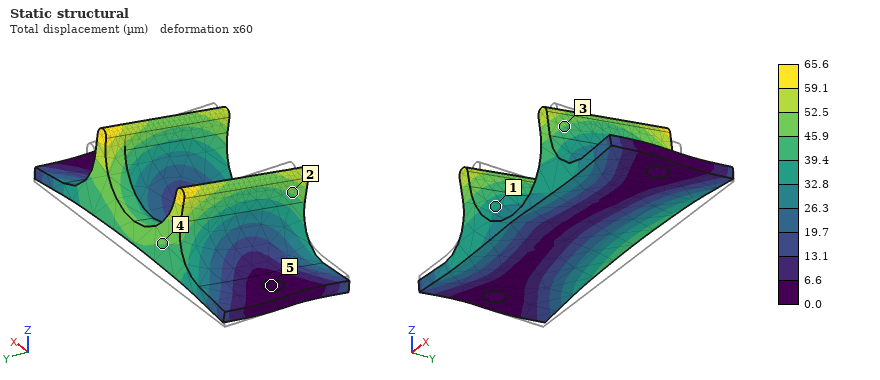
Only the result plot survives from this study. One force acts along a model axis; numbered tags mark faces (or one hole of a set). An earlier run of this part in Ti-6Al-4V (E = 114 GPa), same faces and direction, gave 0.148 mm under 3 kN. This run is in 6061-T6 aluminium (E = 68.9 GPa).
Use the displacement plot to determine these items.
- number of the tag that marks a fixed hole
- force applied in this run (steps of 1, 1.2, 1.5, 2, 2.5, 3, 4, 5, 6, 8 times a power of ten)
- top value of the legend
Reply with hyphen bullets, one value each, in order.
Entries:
- 5
- 800 N
- 65.6 µm
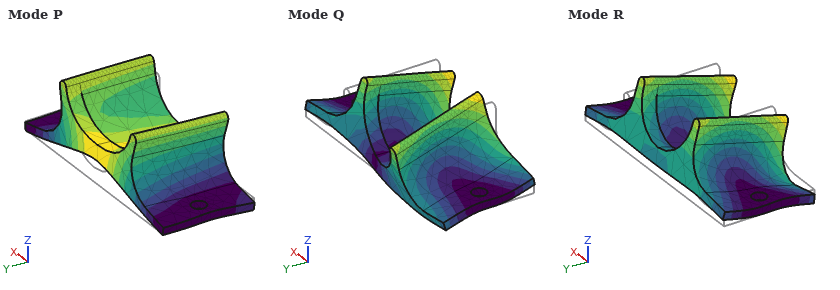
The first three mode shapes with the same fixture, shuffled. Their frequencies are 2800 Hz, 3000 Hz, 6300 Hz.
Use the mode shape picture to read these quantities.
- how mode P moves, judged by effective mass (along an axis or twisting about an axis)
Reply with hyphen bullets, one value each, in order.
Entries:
- along Z
